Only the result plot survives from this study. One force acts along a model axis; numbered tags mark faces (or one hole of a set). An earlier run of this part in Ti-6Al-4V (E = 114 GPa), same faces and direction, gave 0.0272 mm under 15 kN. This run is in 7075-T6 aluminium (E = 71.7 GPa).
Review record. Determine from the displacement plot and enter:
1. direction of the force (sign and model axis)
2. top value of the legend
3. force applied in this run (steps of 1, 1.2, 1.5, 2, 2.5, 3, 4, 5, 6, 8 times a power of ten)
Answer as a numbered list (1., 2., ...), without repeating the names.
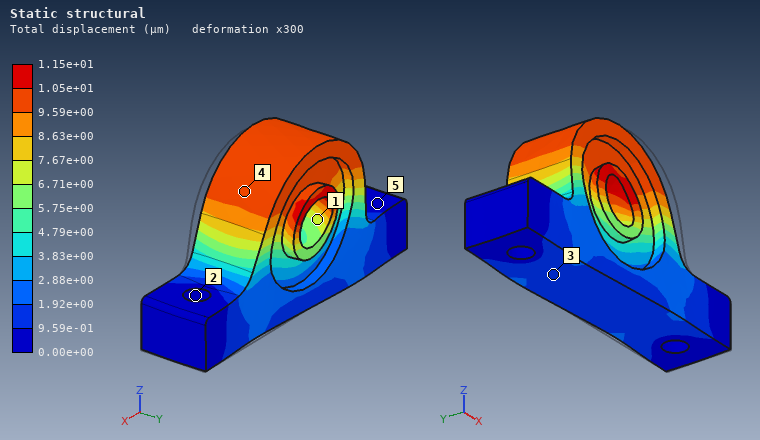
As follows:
1. -X
2. 1.15e+01 µm
3. 4 kN
